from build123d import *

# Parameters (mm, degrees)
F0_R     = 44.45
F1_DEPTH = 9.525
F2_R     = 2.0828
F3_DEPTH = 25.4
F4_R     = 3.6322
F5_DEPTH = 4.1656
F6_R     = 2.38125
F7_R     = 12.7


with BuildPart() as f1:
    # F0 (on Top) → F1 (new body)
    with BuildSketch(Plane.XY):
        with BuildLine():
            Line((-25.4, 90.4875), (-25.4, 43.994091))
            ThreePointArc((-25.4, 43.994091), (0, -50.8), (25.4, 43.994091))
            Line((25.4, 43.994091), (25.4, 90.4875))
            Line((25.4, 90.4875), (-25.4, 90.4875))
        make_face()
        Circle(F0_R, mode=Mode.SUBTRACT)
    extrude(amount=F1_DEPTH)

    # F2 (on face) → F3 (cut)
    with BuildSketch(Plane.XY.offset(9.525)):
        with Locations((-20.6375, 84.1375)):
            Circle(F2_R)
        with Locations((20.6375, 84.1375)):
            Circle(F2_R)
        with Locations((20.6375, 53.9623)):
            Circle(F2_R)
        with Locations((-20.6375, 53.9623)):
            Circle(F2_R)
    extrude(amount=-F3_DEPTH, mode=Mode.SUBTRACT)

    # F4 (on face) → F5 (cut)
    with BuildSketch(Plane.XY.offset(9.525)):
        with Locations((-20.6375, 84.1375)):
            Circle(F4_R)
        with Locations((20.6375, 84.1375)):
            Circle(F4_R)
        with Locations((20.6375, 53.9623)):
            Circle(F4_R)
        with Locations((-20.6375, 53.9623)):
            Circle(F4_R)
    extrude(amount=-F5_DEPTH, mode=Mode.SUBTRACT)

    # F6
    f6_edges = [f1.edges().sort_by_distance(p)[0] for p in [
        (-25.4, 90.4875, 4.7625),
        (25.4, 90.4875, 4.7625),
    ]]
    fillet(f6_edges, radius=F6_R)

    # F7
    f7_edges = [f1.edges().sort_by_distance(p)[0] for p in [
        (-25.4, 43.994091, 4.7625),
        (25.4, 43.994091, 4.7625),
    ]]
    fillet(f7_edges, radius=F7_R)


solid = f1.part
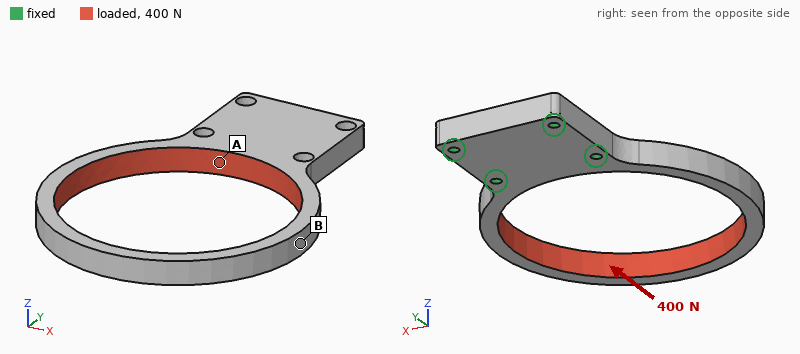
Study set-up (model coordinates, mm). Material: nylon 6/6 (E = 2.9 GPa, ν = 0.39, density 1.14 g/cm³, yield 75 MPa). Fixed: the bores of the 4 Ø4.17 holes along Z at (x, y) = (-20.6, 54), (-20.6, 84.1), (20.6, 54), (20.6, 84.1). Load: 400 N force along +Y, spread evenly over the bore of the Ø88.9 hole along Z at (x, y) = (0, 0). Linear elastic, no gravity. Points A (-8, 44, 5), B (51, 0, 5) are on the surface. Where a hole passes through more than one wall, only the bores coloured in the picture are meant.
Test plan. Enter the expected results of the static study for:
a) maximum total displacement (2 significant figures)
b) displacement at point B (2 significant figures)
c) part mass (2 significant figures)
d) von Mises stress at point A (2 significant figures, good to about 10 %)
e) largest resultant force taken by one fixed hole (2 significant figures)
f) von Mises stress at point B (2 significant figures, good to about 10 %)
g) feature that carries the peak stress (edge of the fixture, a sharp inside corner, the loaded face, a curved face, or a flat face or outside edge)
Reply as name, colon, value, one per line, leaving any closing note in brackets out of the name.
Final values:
maximum total displacement: 2.0 mm
displacement at point B: 1.4 mm
part mass: 43 g
von Mises stress at point A: 3.6 MPa
largest resultant force taken by one fixed hole: 230 N
von Mises stress at point B: 14 MPa
feature that carries the peak stress: a curved face
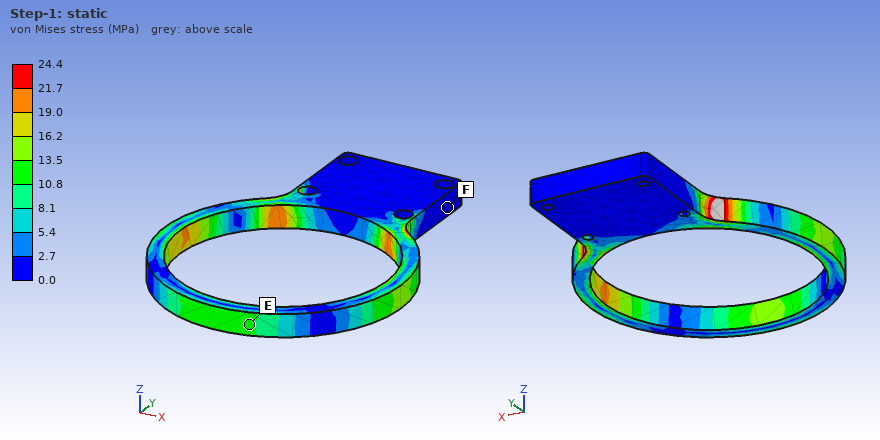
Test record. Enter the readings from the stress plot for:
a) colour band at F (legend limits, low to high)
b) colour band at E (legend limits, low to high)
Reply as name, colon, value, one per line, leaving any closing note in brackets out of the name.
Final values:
colour band at F: 0.0 to 2.7 MPa
colour band at E: 10.8 to 13.5 MPa
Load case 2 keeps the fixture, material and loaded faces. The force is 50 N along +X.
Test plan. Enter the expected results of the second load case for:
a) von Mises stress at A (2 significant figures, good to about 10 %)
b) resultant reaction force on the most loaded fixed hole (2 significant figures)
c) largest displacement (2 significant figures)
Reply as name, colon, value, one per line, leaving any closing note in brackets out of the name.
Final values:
von Mises stress at A: 1.1 MPa
resultant reaction force on the most loaded fixed hole: 64 N
largest displacement: 1.9 mm
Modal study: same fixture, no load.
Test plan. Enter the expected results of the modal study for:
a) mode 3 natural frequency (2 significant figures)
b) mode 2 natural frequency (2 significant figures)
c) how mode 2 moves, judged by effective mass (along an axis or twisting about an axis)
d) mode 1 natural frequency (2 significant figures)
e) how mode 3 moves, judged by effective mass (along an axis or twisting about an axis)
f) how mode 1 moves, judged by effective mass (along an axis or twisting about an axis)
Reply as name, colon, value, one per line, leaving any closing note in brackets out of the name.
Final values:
mode 3 natural frequency: 360 Hz
mode 2 natural frequency: 190 Hz
how mode 2 moves, judged by effective mass: along X
mode 1 natural frequency: 140 Hz
how mode 3 moves, judged by effective mass: twisting about Y
how mode 1 moves, judged by effective mass: along Z
